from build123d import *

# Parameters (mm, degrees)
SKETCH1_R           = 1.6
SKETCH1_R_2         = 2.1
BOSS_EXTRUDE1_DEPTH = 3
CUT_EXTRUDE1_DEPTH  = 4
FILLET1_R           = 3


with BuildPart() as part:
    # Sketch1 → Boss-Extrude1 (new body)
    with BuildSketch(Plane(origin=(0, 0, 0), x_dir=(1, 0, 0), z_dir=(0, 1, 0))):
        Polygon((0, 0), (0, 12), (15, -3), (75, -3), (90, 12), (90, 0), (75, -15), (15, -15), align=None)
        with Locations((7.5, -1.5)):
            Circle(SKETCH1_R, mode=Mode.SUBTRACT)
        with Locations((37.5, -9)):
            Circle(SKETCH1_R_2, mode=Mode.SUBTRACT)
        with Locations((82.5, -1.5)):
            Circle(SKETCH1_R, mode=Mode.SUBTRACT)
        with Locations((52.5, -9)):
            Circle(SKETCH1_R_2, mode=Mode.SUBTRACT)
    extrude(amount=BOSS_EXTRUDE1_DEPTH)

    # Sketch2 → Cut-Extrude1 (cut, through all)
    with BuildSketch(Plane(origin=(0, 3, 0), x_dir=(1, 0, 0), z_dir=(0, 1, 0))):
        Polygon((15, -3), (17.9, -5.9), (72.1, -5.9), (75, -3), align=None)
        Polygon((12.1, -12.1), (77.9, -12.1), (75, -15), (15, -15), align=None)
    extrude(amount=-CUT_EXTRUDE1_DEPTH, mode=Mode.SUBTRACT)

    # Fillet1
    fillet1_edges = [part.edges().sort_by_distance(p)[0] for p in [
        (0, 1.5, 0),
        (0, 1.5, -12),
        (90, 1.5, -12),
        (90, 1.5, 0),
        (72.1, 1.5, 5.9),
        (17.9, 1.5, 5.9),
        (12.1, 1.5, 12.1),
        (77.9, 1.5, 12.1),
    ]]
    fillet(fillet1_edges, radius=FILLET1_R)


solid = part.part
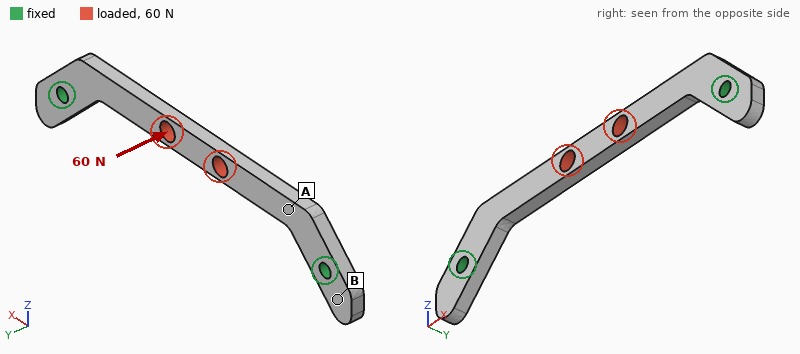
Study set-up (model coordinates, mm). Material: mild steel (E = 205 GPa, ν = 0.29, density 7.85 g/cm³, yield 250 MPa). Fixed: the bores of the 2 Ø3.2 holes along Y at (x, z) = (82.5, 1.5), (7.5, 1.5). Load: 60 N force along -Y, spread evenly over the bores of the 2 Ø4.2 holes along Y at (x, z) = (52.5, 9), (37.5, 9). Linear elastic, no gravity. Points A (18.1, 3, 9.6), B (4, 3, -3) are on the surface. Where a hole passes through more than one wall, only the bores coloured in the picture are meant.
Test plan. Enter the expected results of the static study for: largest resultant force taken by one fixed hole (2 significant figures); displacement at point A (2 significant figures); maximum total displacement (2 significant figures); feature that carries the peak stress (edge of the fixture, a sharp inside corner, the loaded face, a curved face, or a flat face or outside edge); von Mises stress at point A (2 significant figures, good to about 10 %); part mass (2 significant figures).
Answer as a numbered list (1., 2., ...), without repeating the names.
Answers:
1. 30 N
2. 10 µm
3. 49 µm
4. the loaded face
5. 29 MPa
6. 16 g
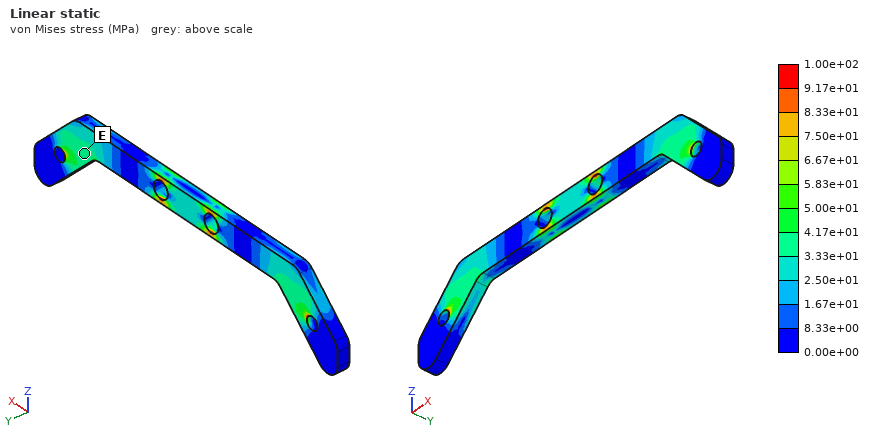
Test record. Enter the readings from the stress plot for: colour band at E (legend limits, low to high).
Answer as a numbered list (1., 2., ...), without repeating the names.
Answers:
1. 3.33e+01 to 4.17e+01 MPa
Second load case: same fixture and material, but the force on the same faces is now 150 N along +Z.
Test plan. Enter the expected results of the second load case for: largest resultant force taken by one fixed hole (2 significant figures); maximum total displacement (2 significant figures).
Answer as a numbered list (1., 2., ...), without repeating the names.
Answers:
1. 140 N
2. 20 µm
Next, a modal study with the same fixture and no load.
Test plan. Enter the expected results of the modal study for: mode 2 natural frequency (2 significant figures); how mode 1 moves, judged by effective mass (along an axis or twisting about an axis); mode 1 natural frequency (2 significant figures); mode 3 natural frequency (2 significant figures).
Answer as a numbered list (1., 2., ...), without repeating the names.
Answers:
1. 7000 Hz
2. along Y
3. 2800 Hz
4. 7100 Hz
